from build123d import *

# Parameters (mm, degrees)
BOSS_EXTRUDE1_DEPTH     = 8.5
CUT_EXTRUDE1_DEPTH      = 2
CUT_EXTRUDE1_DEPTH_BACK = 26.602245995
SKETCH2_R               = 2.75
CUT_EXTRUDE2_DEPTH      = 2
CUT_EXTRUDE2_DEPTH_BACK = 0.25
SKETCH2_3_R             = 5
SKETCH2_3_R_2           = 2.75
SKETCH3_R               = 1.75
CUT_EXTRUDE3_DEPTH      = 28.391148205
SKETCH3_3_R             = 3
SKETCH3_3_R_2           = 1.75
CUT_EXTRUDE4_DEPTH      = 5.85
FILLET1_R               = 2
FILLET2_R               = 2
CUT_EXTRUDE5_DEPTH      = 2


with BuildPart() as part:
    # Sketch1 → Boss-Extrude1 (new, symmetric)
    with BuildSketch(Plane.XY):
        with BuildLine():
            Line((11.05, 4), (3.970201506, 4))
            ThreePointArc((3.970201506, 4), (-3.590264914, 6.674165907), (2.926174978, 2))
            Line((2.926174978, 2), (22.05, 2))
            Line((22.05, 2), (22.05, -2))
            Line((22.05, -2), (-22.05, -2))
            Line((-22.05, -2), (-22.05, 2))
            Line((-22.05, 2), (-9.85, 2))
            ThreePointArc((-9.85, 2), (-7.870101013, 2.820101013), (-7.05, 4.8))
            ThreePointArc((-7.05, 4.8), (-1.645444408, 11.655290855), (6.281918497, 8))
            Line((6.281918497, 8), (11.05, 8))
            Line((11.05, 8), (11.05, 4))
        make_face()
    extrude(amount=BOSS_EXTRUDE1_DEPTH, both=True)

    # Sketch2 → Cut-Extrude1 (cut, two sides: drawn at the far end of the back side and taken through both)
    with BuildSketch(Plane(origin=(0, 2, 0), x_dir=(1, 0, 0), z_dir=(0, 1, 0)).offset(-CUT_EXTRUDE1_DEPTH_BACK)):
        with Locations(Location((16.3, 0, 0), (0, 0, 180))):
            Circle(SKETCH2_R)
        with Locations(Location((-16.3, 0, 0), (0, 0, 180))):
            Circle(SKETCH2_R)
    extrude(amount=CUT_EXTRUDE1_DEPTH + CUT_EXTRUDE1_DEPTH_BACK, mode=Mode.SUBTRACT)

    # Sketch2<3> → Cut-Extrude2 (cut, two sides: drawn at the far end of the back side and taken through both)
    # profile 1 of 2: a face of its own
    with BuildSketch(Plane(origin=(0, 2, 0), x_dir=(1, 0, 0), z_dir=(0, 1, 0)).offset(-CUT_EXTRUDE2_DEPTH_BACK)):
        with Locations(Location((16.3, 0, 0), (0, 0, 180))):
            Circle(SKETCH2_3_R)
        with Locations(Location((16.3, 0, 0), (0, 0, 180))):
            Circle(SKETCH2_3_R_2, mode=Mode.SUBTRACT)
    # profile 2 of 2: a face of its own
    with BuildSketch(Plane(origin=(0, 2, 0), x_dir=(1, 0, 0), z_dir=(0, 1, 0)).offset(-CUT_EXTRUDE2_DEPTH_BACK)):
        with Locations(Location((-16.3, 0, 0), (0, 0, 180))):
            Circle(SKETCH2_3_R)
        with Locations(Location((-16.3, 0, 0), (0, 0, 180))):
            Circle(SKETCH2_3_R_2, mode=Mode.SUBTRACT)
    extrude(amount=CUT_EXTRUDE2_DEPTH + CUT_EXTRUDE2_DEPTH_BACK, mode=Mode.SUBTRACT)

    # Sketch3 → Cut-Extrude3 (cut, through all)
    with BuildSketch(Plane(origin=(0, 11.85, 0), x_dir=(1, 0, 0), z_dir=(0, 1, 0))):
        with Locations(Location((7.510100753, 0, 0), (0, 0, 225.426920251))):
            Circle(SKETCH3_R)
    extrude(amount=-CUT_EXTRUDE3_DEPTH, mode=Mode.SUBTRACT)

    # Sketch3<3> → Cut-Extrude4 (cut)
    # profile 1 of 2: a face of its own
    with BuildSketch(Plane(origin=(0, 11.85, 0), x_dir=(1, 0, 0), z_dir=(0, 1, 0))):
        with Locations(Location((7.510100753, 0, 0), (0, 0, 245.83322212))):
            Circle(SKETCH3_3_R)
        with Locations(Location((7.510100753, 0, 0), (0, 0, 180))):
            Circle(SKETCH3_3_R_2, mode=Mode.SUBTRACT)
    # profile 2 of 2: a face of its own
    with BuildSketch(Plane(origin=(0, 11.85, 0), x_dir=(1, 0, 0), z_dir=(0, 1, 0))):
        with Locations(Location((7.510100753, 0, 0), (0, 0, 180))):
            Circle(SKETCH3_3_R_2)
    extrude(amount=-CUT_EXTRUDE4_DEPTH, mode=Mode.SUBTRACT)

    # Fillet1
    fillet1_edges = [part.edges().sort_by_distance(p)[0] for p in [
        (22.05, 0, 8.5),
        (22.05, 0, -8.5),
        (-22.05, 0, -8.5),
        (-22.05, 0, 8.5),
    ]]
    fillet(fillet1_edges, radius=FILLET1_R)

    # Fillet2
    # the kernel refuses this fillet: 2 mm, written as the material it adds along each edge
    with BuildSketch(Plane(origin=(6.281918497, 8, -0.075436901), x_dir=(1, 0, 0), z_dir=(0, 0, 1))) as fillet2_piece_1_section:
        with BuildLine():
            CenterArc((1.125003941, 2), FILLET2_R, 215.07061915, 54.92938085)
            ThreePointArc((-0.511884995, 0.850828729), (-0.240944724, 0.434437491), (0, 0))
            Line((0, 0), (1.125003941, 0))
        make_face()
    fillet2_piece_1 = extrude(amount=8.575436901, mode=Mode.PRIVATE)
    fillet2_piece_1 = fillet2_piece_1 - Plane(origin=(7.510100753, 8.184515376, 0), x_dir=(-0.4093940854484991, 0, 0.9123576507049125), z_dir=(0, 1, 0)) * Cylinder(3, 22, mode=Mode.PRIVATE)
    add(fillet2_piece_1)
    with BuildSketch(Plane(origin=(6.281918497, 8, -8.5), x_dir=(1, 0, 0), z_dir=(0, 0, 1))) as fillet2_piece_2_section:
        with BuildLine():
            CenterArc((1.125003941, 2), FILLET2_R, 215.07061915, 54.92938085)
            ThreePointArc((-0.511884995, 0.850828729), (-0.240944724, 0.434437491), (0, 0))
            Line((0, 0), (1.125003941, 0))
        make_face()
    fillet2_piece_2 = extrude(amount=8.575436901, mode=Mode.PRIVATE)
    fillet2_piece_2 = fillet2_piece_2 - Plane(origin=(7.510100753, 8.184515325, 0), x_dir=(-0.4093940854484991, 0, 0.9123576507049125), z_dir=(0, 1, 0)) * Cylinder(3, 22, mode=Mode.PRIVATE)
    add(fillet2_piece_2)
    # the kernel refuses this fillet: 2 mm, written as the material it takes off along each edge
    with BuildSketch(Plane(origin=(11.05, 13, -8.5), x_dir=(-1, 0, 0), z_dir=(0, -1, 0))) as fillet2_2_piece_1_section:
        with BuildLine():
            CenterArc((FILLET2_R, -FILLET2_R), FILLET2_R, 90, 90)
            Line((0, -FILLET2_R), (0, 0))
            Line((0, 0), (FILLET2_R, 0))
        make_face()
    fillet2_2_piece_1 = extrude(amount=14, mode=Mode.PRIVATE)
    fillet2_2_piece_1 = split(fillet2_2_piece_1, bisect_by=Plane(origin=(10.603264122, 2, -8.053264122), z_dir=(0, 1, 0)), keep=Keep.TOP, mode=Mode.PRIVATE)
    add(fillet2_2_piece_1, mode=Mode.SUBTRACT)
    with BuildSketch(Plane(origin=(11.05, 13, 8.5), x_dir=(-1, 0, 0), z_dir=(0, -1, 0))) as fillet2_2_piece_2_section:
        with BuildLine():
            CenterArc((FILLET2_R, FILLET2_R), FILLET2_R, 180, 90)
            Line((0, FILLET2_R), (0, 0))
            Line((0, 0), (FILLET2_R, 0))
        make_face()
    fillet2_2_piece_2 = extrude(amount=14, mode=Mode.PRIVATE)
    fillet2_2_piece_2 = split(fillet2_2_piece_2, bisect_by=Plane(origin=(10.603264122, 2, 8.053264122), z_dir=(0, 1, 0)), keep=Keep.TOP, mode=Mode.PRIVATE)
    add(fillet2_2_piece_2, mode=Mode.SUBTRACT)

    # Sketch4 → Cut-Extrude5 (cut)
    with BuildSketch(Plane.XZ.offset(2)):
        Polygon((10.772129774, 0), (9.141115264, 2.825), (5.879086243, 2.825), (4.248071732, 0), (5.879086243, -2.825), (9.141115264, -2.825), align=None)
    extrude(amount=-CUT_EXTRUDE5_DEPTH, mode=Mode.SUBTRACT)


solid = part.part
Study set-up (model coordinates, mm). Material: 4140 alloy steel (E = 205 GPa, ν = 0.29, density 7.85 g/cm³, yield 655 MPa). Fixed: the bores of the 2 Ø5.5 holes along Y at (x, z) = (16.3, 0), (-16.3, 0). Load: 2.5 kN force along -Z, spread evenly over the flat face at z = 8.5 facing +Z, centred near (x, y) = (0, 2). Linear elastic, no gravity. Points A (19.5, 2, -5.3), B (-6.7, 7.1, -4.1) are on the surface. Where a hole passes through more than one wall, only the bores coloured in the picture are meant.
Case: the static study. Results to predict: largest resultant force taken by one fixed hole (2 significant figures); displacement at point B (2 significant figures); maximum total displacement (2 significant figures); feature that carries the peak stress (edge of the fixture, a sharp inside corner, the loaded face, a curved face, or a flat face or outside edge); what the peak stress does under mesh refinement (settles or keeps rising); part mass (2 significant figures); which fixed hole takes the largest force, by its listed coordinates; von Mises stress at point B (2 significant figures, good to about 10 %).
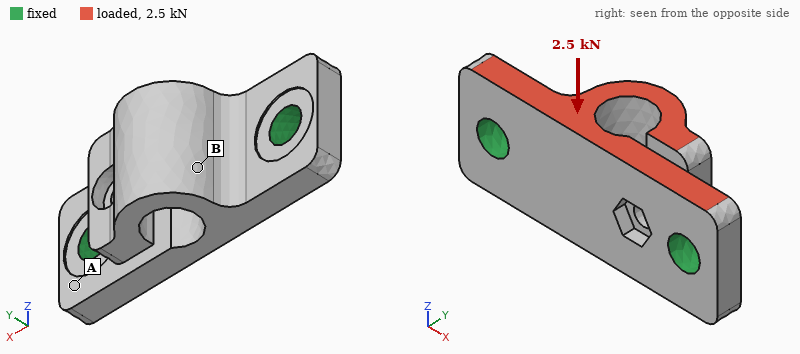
1.3 kN
11 µm
40 µm
edge of the fixture
keeps rising
31 g
(-16.3, 0)
49 MPa
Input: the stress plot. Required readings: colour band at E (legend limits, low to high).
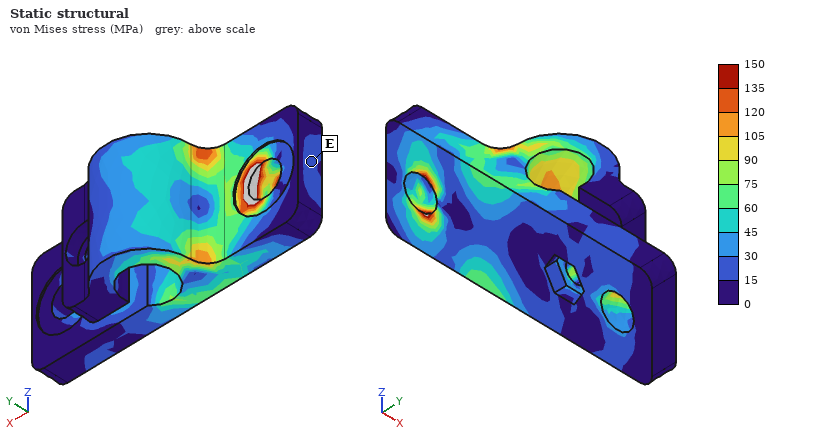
15 to 30 MPa
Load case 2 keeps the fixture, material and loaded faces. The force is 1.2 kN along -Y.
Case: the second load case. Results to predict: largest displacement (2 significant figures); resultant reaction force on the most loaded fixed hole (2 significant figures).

81 µm
630 N
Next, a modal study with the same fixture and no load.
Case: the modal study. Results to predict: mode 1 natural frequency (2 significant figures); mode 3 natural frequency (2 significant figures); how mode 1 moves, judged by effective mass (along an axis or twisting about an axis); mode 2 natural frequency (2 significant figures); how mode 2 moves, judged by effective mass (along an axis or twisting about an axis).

4700 Hz
11 kHz
along Y
7900 Hz
along Z
